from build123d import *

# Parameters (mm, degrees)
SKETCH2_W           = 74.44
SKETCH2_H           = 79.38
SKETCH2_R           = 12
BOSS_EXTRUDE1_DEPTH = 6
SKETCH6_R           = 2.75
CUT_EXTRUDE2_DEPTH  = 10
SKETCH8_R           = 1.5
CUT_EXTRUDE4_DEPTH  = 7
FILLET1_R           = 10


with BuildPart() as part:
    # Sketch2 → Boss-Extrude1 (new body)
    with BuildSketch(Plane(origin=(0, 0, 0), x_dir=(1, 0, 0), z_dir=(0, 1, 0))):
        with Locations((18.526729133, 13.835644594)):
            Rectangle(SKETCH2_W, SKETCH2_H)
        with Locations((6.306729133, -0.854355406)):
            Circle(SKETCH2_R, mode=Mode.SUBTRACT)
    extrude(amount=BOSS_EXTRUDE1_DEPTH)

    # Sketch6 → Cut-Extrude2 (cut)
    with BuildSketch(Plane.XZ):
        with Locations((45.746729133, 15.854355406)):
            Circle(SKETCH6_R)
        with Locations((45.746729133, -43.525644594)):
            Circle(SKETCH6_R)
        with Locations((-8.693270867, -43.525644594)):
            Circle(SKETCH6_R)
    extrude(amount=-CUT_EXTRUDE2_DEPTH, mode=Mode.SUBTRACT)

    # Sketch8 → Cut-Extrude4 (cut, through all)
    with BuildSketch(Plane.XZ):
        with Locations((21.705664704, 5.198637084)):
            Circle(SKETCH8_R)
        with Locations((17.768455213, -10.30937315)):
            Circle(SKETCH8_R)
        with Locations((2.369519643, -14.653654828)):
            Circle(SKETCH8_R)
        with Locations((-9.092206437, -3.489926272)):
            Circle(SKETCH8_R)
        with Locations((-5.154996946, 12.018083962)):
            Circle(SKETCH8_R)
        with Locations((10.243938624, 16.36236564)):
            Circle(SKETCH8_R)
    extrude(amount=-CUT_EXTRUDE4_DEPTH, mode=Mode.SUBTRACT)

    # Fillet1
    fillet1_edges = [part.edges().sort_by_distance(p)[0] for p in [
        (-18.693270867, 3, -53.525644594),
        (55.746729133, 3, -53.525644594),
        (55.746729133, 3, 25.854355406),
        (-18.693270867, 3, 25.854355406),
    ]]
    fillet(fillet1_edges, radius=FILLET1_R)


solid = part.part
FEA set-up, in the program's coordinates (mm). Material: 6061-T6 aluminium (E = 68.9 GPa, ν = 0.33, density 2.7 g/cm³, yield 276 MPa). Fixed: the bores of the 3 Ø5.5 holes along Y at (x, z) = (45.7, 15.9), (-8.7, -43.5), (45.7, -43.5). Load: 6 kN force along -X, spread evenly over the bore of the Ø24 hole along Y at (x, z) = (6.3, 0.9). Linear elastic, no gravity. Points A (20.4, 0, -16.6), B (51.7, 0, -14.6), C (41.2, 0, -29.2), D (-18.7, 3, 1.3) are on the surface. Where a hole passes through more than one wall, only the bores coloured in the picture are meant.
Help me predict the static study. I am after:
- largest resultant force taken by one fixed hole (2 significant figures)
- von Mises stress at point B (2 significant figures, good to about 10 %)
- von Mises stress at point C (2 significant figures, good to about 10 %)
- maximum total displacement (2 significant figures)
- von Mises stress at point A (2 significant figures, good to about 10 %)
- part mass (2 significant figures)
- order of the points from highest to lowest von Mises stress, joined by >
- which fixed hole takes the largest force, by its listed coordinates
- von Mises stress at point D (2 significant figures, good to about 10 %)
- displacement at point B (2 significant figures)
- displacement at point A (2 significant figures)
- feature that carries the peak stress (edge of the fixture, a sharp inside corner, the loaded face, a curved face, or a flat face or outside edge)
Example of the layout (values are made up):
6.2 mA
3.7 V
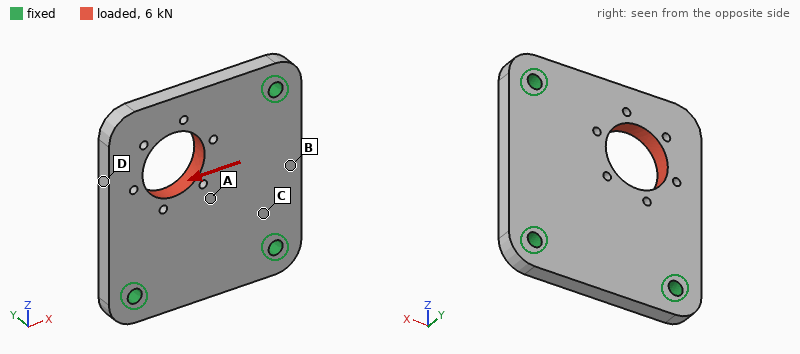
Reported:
3.5 kN
5.6 MPa
12 MPa
26 µm
17 MPa
85 g
D > A > C > B
(45.7, 15.9)
32 MPa
6.7 µm
8.7 µm
a curved face
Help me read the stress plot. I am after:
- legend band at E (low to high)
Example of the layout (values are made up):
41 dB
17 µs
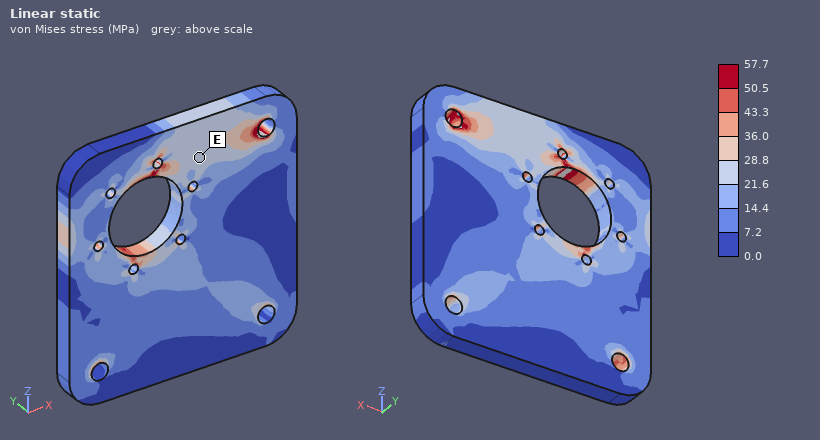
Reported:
21.6 to 28.8 MPa
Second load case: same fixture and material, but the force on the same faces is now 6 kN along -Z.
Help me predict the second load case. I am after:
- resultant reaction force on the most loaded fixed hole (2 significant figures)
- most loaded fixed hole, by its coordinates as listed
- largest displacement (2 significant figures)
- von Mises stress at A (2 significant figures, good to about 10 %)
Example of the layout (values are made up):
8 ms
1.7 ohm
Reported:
3.2 kN
(-8.7, -43.5)
26 µm
12 MPa
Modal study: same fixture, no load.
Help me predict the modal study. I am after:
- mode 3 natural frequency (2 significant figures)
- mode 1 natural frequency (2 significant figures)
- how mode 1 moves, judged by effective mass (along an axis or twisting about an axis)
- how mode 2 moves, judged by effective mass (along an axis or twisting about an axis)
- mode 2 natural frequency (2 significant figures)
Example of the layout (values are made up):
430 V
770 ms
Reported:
6700 Hz
2200 Hz
along Y
along Y
6000 Hz
